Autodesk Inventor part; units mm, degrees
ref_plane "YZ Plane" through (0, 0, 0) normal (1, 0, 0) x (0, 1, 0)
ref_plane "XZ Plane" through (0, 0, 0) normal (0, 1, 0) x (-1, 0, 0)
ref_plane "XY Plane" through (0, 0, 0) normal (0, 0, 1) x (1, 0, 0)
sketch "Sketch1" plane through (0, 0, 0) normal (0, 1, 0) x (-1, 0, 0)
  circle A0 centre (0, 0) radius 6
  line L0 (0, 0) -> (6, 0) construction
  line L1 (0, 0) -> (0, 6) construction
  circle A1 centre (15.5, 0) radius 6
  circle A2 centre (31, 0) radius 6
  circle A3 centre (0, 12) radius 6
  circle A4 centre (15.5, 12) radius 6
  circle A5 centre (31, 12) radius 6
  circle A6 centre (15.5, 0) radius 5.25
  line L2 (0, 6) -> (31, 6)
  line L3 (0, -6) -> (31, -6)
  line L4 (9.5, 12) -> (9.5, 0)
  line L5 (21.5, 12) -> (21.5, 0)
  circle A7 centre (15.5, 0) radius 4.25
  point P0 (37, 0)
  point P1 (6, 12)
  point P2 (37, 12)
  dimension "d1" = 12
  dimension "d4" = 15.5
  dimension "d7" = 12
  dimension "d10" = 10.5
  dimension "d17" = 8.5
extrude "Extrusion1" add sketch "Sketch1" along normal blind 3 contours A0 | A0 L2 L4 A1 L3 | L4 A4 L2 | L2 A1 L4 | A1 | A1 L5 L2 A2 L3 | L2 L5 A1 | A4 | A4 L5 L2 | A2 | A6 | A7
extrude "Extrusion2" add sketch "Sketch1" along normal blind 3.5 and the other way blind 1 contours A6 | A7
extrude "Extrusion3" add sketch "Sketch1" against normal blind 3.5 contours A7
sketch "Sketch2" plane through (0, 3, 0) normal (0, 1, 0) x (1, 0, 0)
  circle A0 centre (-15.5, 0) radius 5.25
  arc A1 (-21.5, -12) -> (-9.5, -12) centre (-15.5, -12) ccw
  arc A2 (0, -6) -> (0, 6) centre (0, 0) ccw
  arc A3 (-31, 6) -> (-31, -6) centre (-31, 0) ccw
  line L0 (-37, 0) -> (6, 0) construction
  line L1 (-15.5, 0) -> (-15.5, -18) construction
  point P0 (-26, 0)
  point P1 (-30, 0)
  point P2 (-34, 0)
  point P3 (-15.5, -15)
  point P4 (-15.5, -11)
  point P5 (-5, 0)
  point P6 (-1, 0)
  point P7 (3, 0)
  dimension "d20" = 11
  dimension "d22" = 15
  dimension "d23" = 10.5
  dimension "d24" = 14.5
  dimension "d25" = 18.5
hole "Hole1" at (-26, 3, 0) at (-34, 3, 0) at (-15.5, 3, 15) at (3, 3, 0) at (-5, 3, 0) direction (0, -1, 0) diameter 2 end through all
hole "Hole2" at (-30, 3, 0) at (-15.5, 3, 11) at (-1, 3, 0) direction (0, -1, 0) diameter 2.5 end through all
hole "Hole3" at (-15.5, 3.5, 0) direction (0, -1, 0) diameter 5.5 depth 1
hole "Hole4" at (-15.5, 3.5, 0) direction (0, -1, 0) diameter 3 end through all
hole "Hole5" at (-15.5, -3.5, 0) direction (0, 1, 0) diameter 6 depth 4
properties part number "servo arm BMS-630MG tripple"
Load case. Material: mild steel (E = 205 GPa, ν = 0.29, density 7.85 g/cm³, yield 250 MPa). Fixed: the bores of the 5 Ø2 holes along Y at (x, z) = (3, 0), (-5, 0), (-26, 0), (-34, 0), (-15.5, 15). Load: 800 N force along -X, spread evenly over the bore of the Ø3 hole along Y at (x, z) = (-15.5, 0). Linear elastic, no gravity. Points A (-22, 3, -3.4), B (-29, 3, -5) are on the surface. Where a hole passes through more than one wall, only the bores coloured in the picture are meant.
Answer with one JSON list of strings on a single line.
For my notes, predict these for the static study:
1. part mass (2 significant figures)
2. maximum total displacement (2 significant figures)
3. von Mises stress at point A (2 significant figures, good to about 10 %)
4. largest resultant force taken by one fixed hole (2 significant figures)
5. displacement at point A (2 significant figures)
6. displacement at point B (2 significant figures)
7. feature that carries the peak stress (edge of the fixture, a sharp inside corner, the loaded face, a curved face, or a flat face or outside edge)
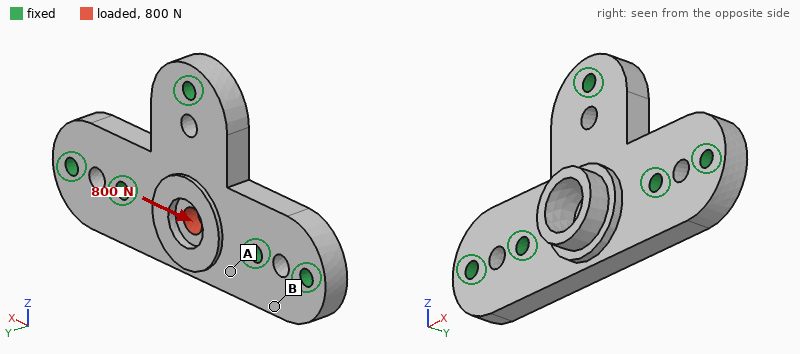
["15 g", "1.0 µm", "10 MPa", "320 N", "0.37 µm", "0.16 µm", "the loaded face"]
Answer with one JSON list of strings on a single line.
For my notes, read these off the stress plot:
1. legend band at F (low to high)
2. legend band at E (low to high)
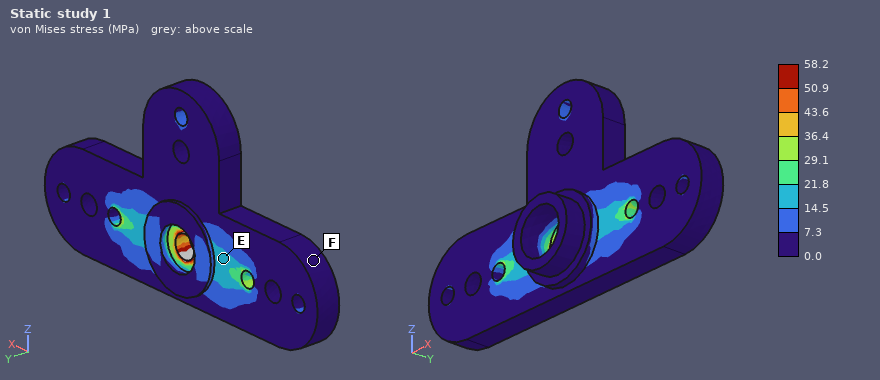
["0.0 to 7.3 MPa", "14.5 to 21.8 MPa"]
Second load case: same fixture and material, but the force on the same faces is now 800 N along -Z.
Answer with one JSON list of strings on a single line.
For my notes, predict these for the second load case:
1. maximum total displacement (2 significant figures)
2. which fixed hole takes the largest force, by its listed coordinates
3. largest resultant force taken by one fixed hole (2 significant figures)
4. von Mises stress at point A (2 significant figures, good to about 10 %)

["1.8 µm", "(-15.5, 15)", "330 N", "13 MPa"]
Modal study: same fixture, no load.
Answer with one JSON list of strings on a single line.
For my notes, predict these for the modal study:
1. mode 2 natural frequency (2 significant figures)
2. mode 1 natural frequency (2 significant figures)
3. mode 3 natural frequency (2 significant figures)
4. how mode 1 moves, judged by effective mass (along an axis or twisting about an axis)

["37 kHz", "29 kHz", "54 kHz", "along Y"]
